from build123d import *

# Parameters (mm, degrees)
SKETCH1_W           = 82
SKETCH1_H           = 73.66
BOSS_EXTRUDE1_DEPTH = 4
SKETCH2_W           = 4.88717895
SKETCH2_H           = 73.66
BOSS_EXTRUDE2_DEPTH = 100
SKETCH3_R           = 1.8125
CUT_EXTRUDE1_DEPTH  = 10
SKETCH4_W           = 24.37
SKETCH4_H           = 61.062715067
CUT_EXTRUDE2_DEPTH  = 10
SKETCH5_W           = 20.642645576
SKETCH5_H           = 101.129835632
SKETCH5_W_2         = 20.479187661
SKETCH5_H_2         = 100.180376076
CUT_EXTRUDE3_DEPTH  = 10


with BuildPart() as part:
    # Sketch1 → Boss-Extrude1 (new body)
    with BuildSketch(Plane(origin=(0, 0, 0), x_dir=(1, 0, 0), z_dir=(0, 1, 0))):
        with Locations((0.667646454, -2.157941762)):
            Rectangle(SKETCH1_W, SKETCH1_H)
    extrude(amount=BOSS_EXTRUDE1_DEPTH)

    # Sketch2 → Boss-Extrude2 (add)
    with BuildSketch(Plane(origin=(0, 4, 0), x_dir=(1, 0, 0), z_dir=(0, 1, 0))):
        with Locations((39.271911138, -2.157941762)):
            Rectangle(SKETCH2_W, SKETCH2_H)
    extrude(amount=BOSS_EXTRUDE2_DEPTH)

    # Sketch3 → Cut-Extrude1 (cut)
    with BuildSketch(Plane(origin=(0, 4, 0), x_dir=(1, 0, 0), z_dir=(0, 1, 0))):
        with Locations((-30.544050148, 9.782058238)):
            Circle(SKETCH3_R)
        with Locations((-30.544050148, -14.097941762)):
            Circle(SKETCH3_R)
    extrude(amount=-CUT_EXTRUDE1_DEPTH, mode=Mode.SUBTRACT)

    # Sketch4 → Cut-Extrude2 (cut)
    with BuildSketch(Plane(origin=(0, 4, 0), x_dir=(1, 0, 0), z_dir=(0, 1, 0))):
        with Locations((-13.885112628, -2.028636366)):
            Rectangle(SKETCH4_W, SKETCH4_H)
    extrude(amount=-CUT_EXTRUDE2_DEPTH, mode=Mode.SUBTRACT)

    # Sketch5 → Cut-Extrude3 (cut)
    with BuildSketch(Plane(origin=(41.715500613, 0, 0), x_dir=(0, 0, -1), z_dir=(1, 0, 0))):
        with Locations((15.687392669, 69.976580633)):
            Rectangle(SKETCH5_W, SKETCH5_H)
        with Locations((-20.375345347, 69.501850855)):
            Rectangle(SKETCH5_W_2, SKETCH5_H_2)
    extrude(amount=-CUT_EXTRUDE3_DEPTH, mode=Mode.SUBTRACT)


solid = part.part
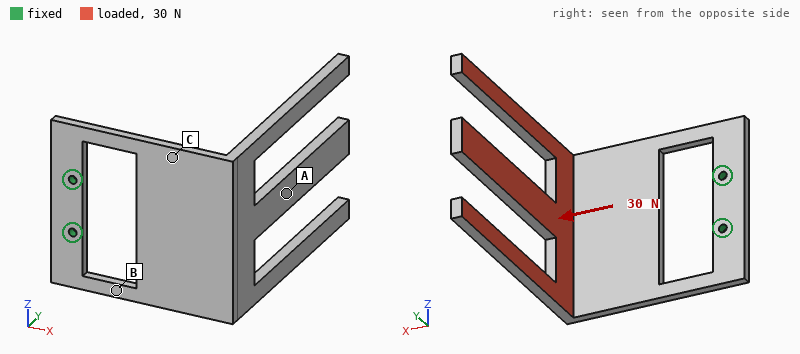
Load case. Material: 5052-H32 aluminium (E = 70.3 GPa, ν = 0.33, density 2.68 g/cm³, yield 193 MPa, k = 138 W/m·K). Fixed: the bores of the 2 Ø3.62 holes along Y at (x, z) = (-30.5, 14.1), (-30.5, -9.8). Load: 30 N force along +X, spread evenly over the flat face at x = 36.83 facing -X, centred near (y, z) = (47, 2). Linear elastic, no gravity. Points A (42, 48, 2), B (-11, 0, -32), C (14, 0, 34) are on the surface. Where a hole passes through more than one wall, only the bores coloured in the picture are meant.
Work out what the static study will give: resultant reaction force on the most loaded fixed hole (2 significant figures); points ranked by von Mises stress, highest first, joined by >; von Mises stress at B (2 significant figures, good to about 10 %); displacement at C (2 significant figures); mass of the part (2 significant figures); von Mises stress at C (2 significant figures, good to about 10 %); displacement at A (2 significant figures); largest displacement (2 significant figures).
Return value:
23 N
B > C > A
40 MPa
0.35 mm
99 g
9.6 MPa
0.95 mm
1.6 mm
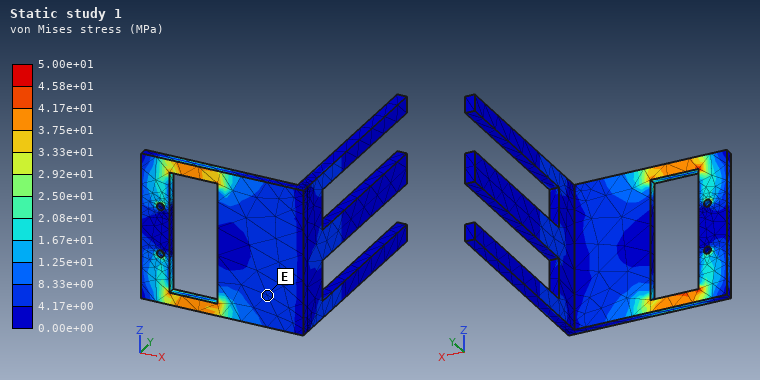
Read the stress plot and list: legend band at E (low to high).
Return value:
4.17e+00 to 8.33e+00 MPa
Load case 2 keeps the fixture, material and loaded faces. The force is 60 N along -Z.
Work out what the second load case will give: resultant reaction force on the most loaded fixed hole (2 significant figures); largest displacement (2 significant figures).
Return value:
130 N
0.84 mm
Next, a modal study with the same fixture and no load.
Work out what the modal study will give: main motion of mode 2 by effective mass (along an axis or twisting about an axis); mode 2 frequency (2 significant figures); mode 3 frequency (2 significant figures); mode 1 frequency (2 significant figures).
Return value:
along Z
220 Hz
380 Hz
87 Hz
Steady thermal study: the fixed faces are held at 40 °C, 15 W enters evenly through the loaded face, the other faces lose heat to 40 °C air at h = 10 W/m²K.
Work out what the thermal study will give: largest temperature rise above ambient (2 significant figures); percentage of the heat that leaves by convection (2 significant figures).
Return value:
71 K
53 %
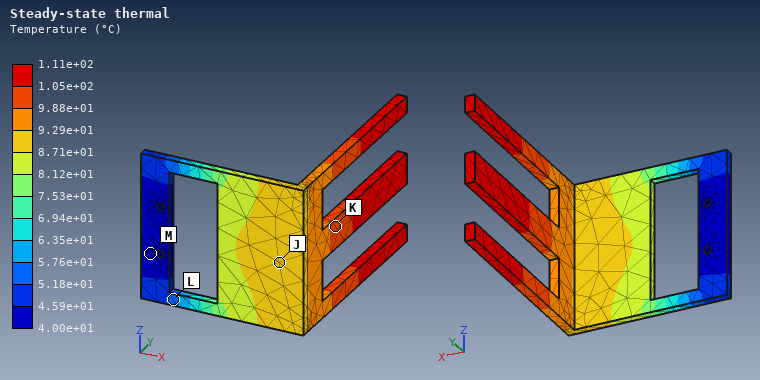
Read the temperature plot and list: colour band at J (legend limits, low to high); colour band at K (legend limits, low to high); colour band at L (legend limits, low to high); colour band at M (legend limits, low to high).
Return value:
8.71e+01 to 9.29e+01 °C
9.88e+01 to 1.05e+02 °C
5.18e+01 to 5.76e+01 °C
4.00e+01 to 4.59e+01 °C
